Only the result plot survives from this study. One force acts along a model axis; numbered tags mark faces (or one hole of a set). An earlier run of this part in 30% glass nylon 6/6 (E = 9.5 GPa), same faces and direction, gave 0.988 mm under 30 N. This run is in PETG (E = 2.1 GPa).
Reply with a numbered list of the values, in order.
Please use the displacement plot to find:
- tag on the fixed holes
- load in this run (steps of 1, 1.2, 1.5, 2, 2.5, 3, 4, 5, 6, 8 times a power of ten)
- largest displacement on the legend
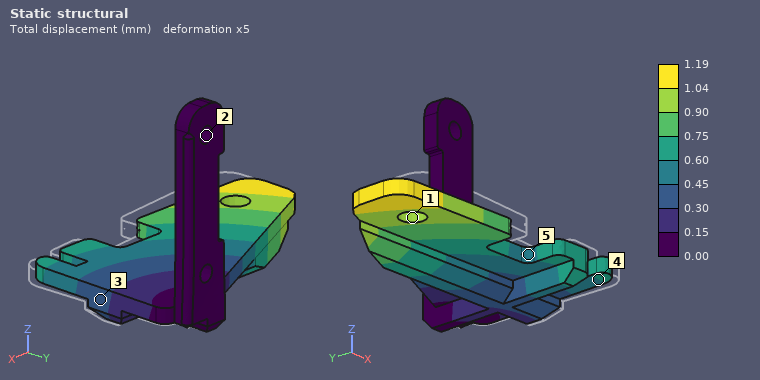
1. 2
2. 8 N
3. 1.19 mm
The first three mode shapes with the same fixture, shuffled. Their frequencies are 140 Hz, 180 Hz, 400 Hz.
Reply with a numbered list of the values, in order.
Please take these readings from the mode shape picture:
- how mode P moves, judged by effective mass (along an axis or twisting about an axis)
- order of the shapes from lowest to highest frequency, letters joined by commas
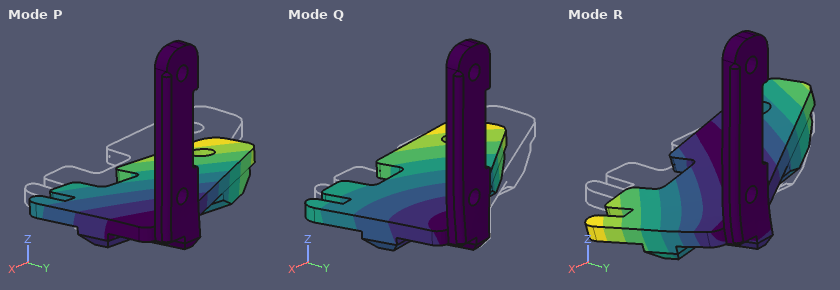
1. along Z
2. P, Q, R
